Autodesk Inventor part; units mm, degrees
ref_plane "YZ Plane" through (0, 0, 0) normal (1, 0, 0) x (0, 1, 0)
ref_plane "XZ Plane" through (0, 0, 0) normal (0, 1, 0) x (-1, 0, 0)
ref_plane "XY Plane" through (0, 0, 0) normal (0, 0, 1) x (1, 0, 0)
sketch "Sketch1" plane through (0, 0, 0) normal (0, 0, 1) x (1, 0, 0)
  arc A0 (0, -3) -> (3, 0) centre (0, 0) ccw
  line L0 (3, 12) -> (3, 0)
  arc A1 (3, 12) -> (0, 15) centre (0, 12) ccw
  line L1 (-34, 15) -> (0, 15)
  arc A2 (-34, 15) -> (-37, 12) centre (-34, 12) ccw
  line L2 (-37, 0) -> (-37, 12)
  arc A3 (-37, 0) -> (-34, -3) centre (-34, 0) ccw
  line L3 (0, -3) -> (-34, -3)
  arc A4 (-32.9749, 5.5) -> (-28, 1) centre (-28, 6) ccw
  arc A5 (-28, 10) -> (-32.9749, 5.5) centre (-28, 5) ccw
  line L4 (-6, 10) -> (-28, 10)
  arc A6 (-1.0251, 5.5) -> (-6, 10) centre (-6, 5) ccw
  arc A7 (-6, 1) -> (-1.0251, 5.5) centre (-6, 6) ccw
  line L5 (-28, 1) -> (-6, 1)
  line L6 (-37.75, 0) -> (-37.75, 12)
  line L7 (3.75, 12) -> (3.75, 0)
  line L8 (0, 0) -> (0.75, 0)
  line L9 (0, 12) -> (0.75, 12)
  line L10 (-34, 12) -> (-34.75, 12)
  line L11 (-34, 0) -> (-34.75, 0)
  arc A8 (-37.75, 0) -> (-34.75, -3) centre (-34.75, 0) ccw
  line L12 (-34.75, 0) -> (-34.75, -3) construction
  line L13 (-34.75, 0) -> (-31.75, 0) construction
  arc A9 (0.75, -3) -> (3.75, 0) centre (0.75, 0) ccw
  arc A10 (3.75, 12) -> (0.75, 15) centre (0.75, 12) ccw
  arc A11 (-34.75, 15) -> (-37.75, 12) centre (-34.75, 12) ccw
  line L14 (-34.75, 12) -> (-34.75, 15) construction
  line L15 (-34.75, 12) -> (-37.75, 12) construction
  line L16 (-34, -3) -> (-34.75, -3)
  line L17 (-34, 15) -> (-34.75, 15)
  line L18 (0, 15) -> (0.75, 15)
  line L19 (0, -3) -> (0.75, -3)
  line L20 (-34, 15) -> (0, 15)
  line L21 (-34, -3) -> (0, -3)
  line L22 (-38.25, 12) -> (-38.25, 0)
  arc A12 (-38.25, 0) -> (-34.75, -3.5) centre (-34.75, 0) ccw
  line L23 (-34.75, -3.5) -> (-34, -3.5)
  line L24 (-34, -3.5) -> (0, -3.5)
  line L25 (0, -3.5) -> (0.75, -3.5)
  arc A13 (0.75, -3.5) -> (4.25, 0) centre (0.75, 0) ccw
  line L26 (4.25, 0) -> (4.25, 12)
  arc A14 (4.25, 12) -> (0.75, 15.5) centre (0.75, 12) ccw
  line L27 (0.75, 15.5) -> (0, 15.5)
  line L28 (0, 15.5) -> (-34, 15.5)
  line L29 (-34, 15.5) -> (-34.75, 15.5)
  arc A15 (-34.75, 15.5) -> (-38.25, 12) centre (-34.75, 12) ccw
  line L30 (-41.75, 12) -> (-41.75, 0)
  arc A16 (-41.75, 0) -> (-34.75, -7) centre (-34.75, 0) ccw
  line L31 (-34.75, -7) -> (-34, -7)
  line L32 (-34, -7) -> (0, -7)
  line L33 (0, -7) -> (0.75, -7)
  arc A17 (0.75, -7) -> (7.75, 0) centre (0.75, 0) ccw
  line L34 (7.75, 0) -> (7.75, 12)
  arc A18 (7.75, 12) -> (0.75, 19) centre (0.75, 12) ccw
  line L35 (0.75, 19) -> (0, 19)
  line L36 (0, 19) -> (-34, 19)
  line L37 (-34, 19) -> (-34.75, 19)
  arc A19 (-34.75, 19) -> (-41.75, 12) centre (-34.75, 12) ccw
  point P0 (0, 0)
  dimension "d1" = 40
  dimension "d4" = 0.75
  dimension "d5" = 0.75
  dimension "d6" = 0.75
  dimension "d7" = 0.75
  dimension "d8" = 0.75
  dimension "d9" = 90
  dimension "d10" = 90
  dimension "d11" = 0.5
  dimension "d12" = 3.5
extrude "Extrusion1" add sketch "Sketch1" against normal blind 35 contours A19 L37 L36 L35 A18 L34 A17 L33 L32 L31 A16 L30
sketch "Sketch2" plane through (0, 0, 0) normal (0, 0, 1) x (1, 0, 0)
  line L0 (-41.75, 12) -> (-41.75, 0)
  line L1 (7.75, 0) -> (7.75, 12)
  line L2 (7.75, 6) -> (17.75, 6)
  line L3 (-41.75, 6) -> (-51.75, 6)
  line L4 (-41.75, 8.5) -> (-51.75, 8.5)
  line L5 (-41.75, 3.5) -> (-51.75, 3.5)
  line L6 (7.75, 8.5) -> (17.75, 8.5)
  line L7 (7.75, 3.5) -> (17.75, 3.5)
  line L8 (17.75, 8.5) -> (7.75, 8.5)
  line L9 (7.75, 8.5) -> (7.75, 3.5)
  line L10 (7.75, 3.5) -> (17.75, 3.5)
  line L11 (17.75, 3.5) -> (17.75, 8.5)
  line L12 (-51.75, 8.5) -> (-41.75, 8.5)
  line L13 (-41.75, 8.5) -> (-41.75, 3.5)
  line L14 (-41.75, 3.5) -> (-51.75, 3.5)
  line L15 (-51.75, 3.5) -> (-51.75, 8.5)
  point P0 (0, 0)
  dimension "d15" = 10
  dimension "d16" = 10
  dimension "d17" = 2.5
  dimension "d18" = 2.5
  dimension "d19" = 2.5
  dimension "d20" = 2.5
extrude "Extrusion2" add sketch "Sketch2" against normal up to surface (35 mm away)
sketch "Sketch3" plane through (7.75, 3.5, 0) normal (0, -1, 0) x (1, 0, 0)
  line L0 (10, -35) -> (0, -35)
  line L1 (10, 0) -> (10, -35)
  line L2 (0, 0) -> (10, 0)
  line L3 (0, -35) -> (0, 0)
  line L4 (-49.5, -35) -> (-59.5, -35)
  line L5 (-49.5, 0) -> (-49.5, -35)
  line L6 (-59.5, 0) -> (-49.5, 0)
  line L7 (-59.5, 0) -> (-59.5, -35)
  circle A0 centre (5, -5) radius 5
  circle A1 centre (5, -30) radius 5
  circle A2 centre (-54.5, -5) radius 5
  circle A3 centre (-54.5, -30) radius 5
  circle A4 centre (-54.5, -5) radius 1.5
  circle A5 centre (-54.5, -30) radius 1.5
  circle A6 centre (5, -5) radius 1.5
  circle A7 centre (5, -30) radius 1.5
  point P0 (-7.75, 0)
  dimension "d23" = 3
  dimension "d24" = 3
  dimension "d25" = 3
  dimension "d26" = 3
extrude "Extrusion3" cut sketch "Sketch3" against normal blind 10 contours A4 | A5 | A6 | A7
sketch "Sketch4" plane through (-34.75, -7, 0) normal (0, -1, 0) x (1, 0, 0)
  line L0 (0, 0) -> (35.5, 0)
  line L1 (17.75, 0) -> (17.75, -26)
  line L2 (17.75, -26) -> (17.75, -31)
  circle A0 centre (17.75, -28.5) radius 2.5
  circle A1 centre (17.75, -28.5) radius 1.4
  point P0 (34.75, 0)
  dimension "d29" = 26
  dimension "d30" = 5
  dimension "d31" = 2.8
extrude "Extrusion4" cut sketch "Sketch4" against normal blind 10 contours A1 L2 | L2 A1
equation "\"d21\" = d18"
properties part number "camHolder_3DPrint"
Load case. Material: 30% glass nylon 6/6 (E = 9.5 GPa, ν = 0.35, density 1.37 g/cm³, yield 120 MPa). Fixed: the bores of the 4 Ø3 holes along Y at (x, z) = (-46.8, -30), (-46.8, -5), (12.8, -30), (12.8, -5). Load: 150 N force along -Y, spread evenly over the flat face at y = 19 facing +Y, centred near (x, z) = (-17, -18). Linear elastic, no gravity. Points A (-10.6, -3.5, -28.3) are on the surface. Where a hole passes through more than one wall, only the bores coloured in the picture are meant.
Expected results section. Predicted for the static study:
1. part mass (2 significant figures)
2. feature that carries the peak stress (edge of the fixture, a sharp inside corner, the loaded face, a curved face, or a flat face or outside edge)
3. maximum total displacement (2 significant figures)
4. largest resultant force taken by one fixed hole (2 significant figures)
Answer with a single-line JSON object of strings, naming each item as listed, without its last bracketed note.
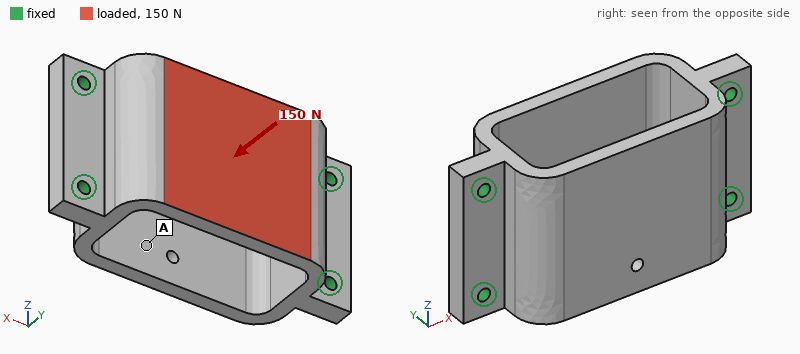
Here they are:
{"part mass": "26 g", "feature that carries the peak stress": "a curved face", "maximum total displacement": "48 µm", "largest resultant force taken by one fixed hole": "58 N"}
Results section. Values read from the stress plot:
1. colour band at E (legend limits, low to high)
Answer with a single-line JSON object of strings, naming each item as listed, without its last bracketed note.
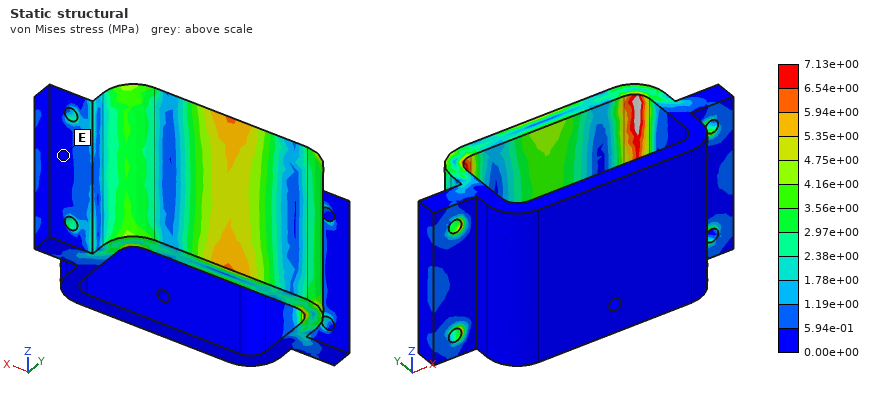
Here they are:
{"colour band at E": "0.00e+00 to 5.94e-01 MPa"}
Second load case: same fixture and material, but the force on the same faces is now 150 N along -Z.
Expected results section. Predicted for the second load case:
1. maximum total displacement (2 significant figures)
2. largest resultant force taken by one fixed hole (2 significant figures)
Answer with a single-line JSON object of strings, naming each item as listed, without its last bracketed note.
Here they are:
{"maximum total displacement": "14 µm", "largest resultant force taken by one fixed hole": "59 N"}
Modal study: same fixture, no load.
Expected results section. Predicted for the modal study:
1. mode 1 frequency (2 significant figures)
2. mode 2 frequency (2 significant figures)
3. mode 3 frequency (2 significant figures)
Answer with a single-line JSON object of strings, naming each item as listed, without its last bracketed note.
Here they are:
{"mode 1 frequency": "4000 Hz", "mode 2 frequency": "4200 Hz", "mode 3 frequency": "4300 Hz"}
